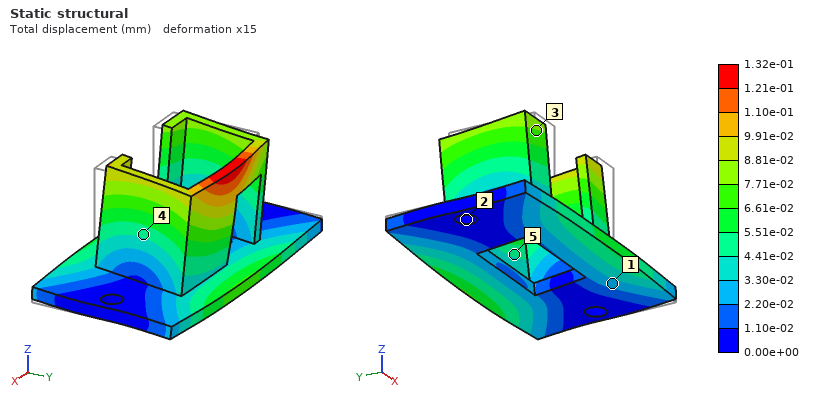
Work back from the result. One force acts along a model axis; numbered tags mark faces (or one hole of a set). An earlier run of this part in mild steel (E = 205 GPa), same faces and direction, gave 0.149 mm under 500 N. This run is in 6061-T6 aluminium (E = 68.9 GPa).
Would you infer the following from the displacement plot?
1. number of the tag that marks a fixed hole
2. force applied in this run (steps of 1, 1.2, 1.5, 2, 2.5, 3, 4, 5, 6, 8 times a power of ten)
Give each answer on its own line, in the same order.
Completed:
2
150 N
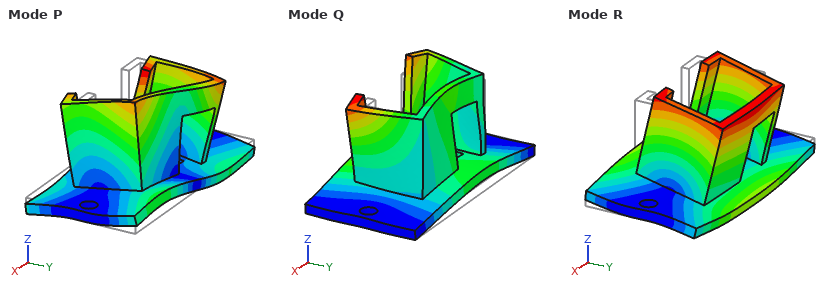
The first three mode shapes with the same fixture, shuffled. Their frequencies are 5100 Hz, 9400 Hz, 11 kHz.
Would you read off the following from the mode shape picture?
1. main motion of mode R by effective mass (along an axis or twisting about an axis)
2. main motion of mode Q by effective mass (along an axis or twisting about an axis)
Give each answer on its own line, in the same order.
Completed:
along Y
along Z
